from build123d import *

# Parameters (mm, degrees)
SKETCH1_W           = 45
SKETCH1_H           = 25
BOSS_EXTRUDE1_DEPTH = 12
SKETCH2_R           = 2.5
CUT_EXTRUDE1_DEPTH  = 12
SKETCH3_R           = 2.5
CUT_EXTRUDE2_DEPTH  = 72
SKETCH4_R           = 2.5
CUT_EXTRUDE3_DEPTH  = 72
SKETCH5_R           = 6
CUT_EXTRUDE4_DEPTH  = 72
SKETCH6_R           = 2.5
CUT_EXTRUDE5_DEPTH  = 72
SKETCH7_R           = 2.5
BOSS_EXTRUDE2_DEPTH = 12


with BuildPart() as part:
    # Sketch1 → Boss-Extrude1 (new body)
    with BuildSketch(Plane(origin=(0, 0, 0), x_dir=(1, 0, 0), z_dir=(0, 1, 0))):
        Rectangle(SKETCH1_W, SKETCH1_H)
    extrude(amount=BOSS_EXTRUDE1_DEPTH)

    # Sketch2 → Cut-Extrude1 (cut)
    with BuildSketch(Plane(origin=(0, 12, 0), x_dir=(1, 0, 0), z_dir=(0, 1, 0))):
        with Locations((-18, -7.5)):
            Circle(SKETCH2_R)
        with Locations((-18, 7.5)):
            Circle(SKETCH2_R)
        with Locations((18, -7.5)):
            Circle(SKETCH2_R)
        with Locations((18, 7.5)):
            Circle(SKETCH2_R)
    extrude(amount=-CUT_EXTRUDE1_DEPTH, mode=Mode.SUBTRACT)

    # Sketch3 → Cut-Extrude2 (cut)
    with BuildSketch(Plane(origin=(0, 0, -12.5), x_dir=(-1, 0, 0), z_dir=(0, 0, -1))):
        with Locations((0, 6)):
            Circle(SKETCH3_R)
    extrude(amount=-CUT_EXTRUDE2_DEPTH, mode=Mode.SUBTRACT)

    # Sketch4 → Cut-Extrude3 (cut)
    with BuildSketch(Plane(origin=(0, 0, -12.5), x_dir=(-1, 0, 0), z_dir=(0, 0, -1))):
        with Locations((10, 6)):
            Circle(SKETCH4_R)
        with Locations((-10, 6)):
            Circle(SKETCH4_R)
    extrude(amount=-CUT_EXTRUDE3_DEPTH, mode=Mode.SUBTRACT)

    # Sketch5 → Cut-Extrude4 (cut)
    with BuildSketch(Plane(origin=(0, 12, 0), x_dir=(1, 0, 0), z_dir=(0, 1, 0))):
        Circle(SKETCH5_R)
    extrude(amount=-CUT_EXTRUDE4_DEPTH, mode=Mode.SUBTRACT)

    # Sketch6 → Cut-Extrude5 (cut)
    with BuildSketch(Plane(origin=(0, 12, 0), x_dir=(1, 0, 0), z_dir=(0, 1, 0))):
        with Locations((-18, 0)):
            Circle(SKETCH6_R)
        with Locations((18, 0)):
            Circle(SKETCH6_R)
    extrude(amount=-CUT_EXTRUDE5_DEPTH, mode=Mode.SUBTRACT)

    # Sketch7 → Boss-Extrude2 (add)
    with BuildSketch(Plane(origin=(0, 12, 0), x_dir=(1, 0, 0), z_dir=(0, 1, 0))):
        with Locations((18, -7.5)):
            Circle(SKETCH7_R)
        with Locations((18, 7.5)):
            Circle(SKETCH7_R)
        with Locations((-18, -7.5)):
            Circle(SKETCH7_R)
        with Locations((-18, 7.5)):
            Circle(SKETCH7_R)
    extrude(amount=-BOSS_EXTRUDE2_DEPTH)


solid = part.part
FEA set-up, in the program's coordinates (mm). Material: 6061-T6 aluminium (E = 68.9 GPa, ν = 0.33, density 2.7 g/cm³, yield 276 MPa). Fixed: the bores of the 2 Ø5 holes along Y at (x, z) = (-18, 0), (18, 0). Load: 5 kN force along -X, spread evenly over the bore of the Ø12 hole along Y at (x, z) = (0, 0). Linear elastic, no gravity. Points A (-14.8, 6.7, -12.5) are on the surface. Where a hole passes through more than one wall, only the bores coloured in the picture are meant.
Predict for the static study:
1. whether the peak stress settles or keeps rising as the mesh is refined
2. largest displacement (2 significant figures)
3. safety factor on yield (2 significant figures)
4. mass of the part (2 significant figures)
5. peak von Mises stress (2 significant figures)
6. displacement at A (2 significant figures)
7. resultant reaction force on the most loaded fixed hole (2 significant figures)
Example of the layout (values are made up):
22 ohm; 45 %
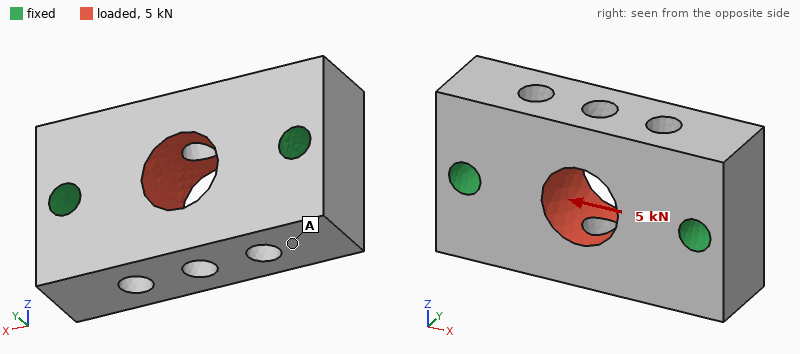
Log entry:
settles; 5.0 µm; 5.0; 28 g; 55 MPa; 2.6 µm; 2.5 kN
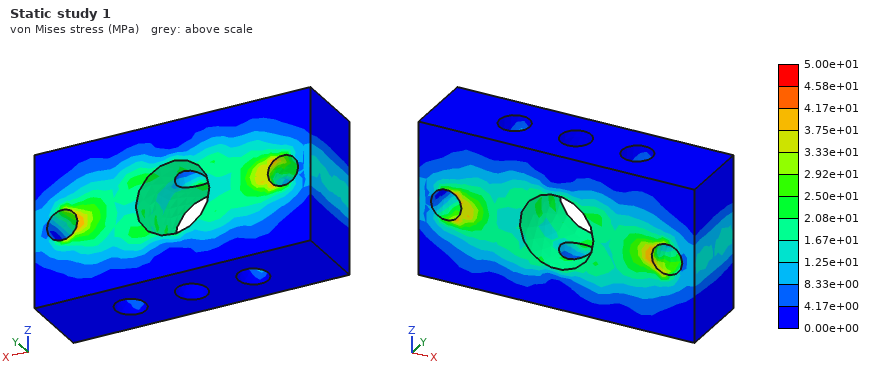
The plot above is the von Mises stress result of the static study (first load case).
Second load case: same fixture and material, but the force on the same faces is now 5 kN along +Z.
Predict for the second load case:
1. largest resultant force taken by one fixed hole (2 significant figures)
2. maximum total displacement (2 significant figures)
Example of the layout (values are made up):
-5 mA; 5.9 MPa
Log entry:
2.5 kN; 12 µm
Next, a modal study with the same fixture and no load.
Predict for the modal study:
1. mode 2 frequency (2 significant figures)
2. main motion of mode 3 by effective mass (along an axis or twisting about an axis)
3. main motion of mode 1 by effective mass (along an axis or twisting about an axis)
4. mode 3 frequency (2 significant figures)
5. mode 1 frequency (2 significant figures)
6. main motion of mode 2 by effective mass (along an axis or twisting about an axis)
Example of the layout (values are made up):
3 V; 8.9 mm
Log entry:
27 kHz; along Z; along Y; 33 kHz; 26 kHz; twisting about X
